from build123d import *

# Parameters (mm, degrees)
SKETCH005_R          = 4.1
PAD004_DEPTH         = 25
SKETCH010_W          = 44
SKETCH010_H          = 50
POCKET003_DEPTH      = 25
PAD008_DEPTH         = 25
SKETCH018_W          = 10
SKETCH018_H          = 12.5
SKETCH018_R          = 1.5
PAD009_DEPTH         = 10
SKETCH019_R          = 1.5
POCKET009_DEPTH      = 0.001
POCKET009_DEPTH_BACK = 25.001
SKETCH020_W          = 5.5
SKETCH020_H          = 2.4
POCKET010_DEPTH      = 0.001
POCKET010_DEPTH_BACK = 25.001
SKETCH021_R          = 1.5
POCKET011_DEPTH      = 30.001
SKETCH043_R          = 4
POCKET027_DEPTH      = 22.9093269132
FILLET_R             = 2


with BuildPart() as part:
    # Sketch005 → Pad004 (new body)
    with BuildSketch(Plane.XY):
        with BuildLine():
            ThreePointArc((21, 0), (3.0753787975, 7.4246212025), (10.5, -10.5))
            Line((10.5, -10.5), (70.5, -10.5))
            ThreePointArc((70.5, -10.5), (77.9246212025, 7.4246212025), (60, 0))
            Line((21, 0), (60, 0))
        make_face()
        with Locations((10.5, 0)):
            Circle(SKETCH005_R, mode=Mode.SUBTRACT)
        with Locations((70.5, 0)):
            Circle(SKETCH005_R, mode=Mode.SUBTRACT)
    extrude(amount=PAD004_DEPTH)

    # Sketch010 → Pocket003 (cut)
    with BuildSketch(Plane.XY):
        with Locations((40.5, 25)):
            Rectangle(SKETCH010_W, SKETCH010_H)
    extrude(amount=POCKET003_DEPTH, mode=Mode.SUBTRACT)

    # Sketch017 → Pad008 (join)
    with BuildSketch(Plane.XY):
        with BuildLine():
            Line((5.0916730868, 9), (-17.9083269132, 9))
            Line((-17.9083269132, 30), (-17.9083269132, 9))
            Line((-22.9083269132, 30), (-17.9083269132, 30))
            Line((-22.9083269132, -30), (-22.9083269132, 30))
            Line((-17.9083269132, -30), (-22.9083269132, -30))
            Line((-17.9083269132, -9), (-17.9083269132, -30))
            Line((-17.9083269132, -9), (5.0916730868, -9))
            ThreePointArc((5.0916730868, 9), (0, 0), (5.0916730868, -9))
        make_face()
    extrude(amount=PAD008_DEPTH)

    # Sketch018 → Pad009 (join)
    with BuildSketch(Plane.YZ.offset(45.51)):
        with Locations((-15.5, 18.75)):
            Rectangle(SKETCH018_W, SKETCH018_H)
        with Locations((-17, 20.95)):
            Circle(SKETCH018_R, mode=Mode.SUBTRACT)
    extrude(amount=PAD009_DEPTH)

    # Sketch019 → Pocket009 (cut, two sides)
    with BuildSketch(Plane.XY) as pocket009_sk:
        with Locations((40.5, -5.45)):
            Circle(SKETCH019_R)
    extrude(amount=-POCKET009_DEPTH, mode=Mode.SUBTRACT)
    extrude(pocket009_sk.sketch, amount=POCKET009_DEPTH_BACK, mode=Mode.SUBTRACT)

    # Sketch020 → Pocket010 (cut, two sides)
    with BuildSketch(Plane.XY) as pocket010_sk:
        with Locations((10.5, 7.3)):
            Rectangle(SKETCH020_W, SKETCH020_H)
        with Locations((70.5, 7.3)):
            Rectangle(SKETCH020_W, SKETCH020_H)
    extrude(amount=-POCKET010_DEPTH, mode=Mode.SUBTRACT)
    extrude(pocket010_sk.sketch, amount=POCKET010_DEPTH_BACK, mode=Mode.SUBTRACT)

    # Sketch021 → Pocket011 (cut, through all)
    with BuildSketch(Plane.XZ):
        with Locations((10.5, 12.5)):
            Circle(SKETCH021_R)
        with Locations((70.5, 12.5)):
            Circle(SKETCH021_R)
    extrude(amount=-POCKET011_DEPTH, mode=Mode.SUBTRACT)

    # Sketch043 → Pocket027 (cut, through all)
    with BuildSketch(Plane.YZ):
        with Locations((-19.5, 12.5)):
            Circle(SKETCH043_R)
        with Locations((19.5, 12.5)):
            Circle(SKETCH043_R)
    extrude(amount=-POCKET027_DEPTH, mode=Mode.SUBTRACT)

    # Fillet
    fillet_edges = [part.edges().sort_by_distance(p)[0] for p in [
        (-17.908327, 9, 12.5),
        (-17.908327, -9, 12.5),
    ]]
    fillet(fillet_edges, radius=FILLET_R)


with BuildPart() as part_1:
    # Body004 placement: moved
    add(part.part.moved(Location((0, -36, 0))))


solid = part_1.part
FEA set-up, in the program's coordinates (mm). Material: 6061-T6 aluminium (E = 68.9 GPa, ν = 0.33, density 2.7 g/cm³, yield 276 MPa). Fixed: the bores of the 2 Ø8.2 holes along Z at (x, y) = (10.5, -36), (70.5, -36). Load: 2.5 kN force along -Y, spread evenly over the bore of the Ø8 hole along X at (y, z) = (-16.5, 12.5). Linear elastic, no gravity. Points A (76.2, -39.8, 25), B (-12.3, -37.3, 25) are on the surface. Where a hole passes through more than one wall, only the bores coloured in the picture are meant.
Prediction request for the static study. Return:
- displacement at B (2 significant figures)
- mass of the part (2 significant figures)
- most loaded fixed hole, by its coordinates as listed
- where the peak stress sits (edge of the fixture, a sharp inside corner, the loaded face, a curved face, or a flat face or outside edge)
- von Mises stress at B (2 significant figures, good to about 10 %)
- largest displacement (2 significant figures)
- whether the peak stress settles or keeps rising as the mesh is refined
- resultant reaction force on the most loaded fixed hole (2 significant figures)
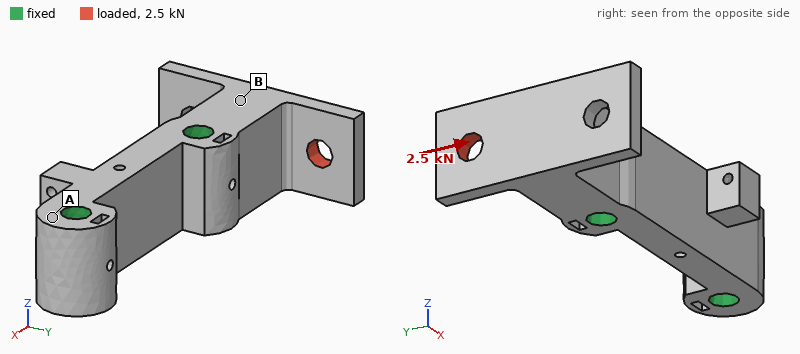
27 µm
110 g
(10.5, -36)
edge of the fixture
19 MPa
82 µm
keeps rising
2.7 kN
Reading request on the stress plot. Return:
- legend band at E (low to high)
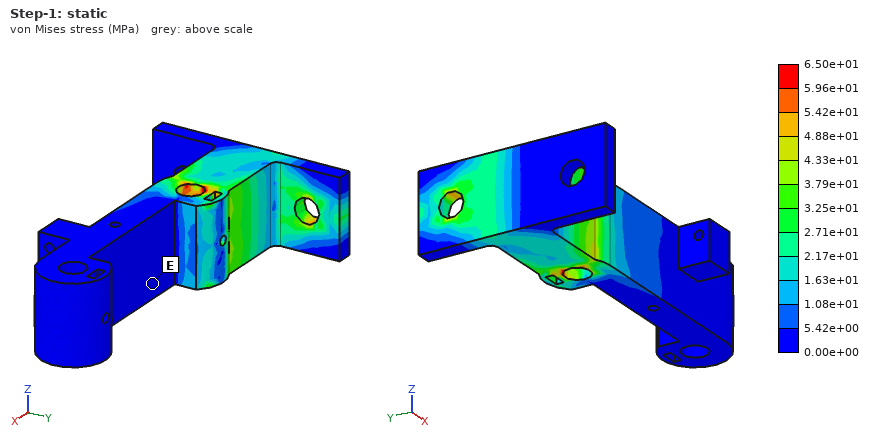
0.00e+00 to 5.42e+00 MPa
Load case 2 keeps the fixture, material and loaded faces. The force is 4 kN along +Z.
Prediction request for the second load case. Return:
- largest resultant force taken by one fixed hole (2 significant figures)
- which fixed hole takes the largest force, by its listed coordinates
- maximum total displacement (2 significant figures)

4.1 kN
(10.5, -36)
0.18 mm
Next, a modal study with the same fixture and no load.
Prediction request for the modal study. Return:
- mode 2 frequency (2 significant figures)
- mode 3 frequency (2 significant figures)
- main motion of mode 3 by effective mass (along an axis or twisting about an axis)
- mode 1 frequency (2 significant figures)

7400 Hz
8800 Hz
twisting about X
5600 Hz
